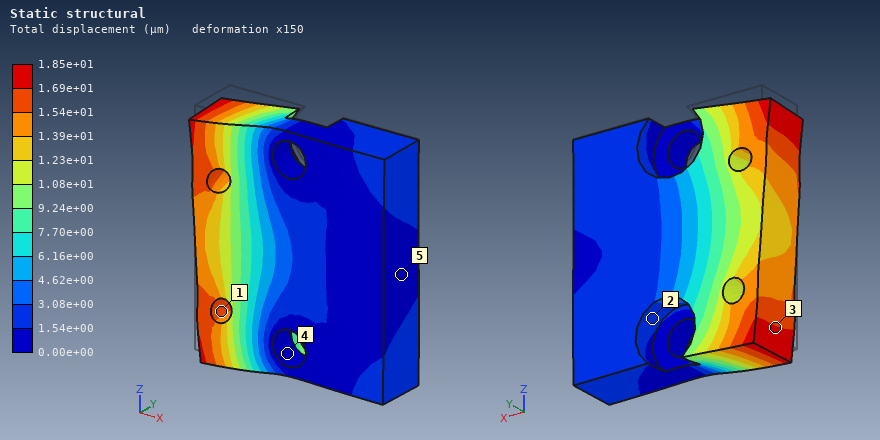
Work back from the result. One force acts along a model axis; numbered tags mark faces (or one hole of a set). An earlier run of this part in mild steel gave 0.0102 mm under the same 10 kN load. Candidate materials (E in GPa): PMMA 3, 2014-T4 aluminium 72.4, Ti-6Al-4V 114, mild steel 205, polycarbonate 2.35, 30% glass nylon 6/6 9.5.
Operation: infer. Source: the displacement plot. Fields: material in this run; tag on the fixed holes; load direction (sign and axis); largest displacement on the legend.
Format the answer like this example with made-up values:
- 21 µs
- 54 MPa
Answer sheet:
- Ti-6Al-4V
- 4
- -Z
- 1.85e+01 µm
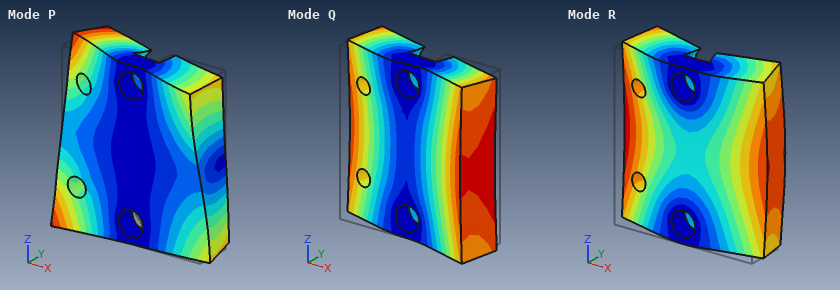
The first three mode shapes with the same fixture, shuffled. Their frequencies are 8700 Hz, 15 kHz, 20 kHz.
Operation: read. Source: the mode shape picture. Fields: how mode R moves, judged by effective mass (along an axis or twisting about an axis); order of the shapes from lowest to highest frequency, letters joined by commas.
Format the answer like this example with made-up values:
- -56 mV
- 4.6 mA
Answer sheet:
- along Y
- Q, R, P
